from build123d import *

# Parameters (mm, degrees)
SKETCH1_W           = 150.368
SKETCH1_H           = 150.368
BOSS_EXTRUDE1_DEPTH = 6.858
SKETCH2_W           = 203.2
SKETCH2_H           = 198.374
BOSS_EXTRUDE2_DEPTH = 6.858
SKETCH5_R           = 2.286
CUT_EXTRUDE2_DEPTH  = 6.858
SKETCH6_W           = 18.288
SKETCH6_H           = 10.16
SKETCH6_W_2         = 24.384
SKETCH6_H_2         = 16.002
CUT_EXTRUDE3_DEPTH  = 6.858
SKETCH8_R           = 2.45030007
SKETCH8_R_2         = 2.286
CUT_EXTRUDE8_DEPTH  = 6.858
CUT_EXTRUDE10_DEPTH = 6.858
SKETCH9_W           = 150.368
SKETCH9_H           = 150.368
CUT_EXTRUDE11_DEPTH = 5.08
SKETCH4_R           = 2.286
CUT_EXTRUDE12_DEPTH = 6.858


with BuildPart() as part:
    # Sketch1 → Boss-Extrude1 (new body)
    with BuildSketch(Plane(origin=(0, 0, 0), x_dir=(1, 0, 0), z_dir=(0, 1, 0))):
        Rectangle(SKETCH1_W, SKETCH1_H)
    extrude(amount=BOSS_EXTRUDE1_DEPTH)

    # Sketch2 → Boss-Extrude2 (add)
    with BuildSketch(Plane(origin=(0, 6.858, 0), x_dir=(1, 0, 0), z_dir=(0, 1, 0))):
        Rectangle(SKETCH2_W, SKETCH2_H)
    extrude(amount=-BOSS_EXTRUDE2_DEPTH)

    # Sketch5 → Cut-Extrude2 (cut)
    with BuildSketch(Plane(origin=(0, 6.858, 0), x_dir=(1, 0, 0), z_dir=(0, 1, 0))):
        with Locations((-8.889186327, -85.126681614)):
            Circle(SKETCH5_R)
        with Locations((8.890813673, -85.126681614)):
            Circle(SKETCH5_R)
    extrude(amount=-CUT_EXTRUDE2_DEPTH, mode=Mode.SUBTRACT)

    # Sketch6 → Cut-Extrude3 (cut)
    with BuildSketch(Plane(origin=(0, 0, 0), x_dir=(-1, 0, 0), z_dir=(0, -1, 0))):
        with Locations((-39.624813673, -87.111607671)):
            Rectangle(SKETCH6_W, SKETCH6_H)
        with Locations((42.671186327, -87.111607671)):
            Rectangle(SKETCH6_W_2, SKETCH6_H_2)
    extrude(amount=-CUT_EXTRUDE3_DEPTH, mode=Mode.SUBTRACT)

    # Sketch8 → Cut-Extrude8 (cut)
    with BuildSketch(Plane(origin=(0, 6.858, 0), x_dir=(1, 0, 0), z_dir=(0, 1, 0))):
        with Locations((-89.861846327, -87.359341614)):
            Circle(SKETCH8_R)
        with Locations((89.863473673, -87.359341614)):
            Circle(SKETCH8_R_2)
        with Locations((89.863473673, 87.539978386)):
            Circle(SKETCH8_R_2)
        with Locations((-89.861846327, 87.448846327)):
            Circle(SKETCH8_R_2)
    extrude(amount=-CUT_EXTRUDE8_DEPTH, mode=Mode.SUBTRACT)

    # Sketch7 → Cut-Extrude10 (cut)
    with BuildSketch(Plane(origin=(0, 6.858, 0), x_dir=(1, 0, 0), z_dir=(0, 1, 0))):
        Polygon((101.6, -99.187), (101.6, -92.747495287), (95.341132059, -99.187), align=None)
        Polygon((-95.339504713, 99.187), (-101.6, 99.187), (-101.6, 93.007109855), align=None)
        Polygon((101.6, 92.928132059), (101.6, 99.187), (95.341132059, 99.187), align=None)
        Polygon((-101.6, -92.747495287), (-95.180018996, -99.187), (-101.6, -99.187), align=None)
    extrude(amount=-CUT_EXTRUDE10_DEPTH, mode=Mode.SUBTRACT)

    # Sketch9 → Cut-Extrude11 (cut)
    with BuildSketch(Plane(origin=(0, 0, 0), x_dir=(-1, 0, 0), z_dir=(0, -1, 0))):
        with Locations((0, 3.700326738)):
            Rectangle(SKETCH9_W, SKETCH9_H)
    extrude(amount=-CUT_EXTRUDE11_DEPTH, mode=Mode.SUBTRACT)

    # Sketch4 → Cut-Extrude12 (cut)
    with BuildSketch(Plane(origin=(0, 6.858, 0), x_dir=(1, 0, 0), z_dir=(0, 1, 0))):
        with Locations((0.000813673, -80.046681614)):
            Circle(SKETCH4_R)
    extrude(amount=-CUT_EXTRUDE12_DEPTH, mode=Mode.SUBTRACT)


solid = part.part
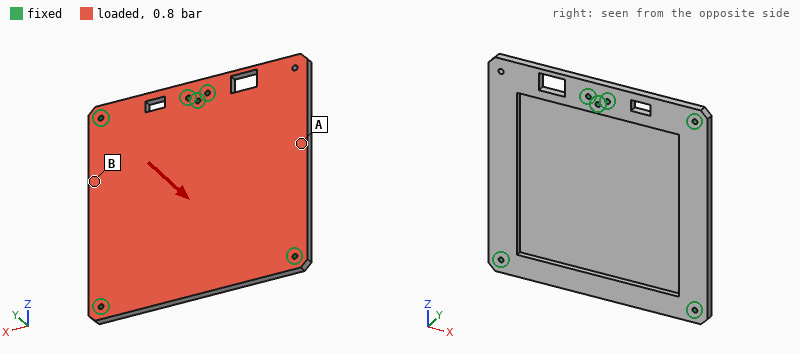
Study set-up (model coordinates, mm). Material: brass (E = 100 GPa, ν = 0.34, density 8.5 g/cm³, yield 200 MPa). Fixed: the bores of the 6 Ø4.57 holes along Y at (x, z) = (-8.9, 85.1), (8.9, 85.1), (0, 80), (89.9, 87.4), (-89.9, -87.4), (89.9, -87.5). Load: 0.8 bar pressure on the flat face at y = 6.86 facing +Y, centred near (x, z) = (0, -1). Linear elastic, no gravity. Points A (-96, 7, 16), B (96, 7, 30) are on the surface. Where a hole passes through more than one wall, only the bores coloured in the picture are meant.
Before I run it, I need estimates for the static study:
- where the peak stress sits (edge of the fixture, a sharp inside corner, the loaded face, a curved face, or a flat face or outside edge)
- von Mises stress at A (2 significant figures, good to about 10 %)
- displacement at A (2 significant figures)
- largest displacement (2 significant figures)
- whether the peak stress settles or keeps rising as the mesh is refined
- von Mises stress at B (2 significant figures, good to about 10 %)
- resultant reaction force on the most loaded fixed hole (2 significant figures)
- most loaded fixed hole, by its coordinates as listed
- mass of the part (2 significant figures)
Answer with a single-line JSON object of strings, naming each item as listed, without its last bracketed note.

{"where the peak stress sits": "edge of the fixture", "von Mises stress at A": "43 MPa", "displacement at A": "0.49 mm", "largest displacement": "1.3 mm", "whether the peak stress settles or keeps rising as the mesh is refined": "keeps rising", "von Mises stress at B": "19 MPa", "resultant reaction force on the most loaded fixed hole": "2.0 kN", "most loaded fixed hole, by its coordinates as listed": "(-89.9, -87.4)", "mass of the part": "1.3 kg"}
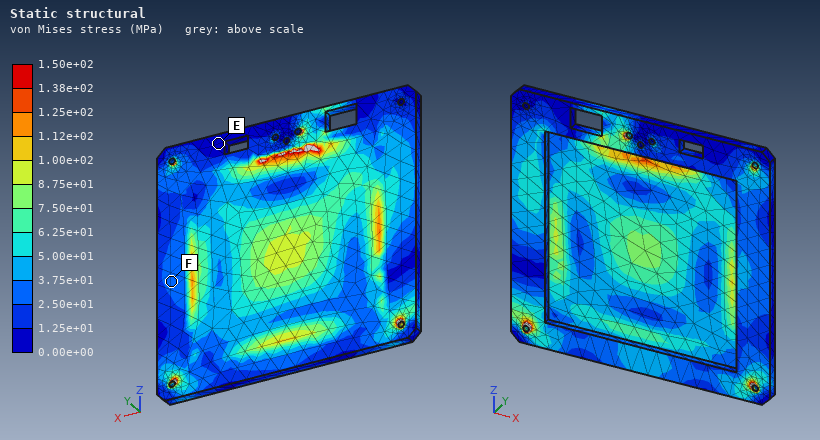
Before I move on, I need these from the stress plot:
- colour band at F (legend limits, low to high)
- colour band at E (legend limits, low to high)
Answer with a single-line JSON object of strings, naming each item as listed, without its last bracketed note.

{"colour band at F": "2.50e+01 to 3.75e+01 MPa", "colour band at E": "0.00e+00 to 1.25e+01 MPa"}
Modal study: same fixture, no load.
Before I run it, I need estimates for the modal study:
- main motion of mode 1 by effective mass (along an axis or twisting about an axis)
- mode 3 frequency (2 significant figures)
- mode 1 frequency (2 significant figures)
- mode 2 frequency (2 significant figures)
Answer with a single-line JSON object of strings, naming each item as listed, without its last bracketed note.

{"main motion of mode 1 by effective mass": "along Y", "mode 3 frequency": "680 Hz", "mode 1 frequency": "350 Hz", "mode 2 frequency": "420 Hz"}
